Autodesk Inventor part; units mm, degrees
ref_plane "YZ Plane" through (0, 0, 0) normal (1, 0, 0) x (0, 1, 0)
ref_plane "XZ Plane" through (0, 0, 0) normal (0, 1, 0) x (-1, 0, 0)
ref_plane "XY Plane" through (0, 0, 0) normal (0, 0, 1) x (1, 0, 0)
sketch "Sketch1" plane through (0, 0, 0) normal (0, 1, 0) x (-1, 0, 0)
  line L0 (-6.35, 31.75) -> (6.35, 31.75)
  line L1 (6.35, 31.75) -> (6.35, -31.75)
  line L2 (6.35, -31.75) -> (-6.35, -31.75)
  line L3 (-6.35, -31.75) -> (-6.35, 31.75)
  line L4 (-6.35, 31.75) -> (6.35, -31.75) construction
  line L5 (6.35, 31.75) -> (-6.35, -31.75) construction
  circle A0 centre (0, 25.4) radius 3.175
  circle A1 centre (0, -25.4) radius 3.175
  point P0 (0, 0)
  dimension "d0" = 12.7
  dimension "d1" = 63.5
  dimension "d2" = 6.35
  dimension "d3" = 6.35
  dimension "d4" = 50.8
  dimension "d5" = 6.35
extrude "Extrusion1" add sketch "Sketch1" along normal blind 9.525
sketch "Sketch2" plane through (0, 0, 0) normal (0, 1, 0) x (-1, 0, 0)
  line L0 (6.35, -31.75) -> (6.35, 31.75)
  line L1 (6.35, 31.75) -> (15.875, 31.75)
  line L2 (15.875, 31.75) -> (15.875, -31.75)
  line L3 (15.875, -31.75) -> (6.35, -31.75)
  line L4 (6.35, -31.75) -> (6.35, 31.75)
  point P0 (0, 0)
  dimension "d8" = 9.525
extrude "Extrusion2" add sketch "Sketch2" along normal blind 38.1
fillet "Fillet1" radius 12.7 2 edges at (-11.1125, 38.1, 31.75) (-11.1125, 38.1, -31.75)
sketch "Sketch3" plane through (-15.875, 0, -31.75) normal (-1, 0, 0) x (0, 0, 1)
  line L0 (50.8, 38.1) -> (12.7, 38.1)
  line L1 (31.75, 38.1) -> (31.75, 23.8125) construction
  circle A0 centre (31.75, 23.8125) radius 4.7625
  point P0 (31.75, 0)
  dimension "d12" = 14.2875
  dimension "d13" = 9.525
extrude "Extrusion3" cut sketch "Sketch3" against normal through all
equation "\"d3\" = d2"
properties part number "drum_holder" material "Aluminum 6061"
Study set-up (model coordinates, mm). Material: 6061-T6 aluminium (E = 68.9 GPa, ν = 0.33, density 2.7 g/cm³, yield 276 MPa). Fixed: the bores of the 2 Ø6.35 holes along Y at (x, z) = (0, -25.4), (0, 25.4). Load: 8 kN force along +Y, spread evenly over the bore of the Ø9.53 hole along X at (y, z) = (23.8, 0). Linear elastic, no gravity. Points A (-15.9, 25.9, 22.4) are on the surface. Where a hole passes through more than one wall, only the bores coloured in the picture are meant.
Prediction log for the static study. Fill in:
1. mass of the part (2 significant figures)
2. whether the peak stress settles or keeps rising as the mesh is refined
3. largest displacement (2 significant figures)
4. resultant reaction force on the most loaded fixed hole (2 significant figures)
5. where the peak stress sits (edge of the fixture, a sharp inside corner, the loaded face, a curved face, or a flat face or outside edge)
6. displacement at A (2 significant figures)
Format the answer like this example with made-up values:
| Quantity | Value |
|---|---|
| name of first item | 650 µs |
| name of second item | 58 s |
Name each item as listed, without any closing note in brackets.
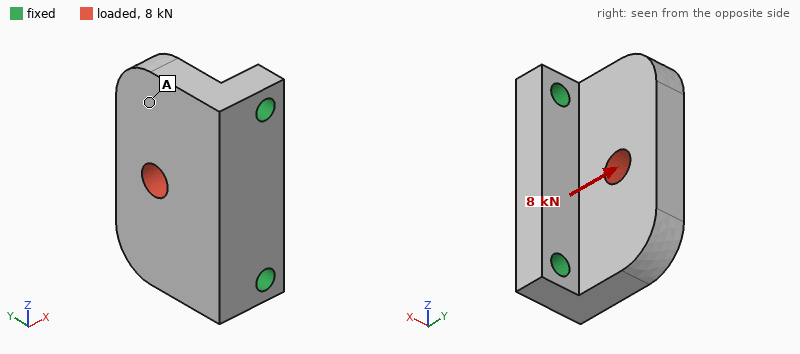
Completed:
| Quantity | Value |
|---|---|
| mass of the part | 78 g |
| whether the peak stress settles or keeps rising as the mesh is refined | keeps rising |
| largest displacement | 0.11 mm |
| resultant reaction force on the most loaded fixed hole | 4.1 kN |
| where the peak stress sits | edge of the fixture |
| displacement at A | 0.070 mm |
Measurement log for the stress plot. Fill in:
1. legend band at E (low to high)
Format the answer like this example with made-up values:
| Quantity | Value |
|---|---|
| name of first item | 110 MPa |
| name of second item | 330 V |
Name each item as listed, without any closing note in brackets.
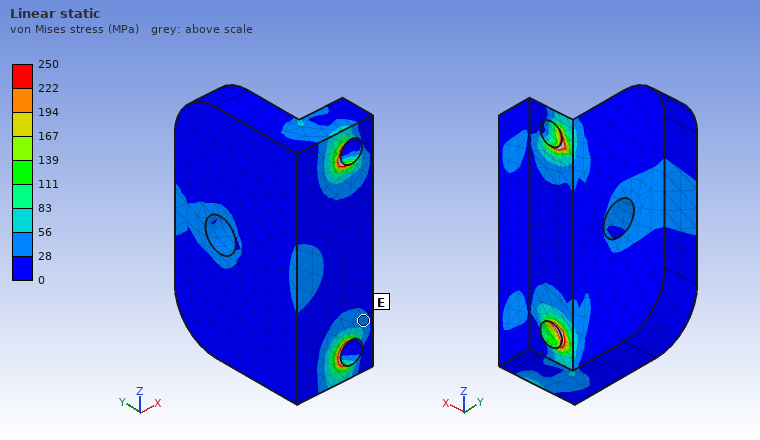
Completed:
| Quantity | Value |
|---|---|
| legend band at E | 28 to 56 MPa |
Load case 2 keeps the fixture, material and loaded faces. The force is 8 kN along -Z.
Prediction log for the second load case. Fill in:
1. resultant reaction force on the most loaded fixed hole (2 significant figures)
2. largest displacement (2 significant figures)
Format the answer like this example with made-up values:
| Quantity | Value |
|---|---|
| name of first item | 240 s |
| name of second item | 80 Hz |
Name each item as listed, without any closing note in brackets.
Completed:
| Quantity | Value |
|---|---|
| resultant reaction force on the most loaded fixed hole | 5.2 kN |
| largest displacement | 42 µm |
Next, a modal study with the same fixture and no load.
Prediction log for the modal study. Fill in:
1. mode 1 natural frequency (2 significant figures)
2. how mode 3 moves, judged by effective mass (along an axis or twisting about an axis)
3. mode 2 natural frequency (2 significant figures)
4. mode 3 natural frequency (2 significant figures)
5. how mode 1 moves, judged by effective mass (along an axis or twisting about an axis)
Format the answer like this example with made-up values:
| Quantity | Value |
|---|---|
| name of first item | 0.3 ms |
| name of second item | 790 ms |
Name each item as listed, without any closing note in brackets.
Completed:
| Quantity | Value |
|---|---|
| mode 1 natural frequency | 4400 Hz |
| how mode 3 moves, judged by effective mass | along Z |
| mode 2 natural frequency | 8800 Hz |
| mode 3 natural frequency | 13 kHz |
| how mode 1 moves, judged by effective mass | along X |
